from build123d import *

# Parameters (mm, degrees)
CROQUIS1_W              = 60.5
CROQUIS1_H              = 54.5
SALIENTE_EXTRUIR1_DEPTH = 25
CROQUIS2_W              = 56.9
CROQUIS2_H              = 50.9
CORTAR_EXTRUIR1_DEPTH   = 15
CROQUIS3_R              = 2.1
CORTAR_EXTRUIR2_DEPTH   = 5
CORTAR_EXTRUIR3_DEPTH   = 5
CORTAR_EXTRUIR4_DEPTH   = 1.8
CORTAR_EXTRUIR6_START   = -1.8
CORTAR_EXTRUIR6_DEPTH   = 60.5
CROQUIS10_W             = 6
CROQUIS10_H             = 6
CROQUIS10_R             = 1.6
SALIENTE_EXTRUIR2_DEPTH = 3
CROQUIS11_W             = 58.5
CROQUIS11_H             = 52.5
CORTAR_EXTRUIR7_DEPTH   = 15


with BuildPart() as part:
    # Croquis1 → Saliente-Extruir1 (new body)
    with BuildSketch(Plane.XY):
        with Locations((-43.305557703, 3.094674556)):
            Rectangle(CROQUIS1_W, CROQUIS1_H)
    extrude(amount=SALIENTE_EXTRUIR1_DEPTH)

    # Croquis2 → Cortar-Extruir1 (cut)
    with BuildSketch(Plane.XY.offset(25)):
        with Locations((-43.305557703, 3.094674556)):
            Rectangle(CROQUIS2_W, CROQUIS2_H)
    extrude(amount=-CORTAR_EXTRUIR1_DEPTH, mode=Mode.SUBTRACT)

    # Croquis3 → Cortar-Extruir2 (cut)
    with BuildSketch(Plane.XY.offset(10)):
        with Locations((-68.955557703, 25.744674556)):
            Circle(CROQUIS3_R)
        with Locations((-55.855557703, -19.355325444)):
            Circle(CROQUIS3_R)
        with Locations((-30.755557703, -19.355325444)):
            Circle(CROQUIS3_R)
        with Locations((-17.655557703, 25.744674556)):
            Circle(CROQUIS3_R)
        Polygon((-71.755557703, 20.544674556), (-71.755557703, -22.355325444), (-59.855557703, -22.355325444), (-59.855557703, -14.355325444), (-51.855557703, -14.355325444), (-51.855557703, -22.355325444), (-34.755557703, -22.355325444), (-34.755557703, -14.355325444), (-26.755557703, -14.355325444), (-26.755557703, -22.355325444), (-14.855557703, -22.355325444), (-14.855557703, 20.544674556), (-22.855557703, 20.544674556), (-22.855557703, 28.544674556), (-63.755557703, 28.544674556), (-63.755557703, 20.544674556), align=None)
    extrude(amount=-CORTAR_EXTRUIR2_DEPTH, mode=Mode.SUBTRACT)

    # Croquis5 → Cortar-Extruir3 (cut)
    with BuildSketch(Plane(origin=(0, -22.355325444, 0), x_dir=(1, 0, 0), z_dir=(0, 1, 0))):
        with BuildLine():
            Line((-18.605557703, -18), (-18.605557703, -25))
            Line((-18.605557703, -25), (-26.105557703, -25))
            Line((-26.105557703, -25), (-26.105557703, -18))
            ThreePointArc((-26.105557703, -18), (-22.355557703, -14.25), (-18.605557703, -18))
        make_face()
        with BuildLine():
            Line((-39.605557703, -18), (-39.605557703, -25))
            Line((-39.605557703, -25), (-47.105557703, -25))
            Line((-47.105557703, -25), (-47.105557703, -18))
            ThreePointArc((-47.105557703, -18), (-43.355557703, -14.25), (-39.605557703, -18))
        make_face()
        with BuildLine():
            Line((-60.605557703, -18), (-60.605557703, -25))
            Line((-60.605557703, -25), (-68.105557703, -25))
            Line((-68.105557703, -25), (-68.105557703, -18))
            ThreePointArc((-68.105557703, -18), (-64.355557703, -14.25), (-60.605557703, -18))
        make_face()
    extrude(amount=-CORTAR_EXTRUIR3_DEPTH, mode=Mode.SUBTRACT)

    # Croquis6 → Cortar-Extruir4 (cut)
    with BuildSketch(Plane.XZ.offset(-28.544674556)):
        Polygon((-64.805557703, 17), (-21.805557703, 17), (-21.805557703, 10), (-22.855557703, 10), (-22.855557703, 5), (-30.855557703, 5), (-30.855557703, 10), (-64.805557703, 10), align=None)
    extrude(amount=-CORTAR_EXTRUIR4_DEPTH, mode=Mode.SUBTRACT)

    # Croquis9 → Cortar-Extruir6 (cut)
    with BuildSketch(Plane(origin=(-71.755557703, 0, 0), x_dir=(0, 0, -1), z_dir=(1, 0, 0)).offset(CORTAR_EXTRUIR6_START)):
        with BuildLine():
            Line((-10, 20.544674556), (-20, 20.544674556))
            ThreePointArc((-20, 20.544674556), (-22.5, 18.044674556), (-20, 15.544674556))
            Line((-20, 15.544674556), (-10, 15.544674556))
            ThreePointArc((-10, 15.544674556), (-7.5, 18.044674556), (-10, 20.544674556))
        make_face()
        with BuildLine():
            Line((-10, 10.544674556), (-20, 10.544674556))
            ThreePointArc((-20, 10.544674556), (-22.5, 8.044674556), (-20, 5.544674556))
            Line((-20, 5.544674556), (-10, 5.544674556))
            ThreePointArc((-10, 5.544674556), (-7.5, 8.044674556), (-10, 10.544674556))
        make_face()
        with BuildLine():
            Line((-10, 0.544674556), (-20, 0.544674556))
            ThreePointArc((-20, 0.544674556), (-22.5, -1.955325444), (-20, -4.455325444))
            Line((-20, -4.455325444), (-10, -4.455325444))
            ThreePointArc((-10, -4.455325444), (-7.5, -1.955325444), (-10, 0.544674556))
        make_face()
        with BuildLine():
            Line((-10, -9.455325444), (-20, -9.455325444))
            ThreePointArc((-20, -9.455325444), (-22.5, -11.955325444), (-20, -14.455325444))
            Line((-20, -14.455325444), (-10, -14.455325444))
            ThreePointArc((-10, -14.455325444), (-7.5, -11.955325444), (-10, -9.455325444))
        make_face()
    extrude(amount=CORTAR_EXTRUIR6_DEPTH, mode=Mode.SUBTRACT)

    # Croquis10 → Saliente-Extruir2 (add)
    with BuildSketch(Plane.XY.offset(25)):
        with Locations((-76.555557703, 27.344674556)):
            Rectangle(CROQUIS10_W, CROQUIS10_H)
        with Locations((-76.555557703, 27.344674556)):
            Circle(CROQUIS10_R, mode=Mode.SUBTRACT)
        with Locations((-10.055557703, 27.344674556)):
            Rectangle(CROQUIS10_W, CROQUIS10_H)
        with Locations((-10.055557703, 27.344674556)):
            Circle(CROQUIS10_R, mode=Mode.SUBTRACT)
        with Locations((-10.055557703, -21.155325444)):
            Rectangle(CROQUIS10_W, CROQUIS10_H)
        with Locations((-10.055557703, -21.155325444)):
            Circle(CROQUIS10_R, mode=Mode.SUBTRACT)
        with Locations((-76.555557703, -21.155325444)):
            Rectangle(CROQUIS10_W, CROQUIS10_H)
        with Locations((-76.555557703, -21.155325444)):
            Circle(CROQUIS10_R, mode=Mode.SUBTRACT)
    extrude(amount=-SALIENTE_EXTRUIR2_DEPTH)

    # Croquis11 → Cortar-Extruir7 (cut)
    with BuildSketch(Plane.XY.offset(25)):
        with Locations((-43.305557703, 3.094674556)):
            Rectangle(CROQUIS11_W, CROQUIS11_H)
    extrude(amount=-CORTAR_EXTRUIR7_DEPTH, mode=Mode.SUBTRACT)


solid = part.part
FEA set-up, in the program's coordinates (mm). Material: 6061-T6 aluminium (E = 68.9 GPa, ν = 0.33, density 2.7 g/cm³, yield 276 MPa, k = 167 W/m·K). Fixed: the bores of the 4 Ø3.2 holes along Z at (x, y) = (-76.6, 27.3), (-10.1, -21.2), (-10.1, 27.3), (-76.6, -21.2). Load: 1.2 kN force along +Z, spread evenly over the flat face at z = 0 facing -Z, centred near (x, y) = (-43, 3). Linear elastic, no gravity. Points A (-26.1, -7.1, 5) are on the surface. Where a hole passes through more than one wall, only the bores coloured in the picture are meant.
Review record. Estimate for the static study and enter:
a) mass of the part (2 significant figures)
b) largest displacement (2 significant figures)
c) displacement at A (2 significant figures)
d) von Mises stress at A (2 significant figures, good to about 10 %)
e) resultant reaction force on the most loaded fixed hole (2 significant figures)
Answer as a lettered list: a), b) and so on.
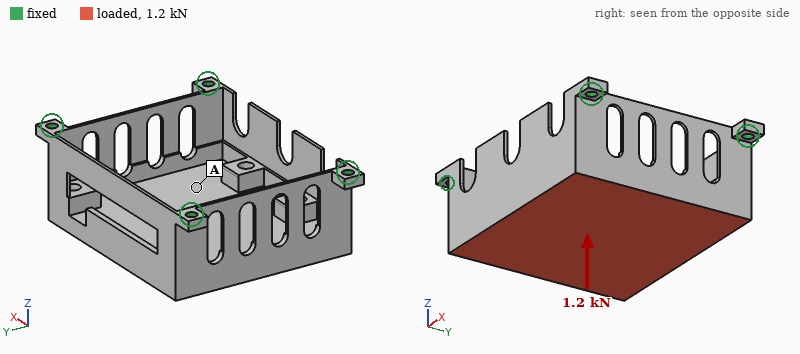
a) 59 g
b) 38 µm
c) 26 µm
d) 9.7 MPa
e) 310 N
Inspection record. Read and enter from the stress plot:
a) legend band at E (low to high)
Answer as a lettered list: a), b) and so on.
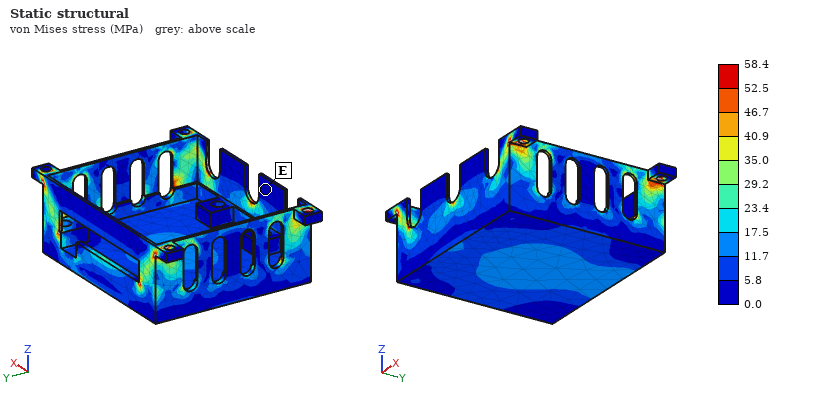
a) 0.0 to 5.8 MPa
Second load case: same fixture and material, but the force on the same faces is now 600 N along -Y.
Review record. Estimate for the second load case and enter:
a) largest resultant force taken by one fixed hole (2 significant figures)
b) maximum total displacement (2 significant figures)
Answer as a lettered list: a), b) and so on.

a) 200 N
b) 25 µm
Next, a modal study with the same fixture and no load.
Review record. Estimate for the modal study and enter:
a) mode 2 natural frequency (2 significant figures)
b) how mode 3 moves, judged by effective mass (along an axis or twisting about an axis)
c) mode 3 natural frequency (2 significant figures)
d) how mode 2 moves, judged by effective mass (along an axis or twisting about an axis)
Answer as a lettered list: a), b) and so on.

a) 2900 Hz
b) along Y
c) 3400 Hz
d) along X
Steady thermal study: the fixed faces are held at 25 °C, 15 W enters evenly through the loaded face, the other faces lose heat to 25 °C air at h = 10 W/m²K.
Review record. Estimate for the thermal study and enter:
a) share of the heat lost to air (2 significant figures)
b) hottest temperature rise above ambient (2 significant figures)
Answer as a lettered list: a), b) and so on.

a) 14 %
b) 22 K
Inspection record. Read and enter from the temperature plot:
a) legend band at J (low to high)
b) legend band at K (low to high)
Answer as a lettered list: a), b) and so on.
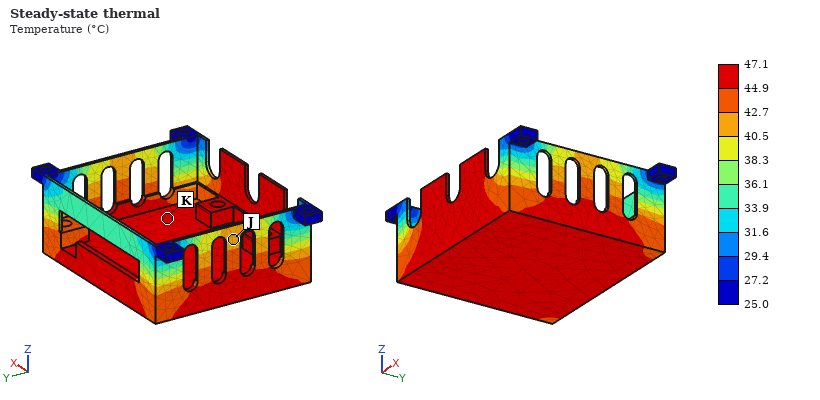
a) 40.5 to 42.7 °C
b) 44.9 to 47.1 °C
